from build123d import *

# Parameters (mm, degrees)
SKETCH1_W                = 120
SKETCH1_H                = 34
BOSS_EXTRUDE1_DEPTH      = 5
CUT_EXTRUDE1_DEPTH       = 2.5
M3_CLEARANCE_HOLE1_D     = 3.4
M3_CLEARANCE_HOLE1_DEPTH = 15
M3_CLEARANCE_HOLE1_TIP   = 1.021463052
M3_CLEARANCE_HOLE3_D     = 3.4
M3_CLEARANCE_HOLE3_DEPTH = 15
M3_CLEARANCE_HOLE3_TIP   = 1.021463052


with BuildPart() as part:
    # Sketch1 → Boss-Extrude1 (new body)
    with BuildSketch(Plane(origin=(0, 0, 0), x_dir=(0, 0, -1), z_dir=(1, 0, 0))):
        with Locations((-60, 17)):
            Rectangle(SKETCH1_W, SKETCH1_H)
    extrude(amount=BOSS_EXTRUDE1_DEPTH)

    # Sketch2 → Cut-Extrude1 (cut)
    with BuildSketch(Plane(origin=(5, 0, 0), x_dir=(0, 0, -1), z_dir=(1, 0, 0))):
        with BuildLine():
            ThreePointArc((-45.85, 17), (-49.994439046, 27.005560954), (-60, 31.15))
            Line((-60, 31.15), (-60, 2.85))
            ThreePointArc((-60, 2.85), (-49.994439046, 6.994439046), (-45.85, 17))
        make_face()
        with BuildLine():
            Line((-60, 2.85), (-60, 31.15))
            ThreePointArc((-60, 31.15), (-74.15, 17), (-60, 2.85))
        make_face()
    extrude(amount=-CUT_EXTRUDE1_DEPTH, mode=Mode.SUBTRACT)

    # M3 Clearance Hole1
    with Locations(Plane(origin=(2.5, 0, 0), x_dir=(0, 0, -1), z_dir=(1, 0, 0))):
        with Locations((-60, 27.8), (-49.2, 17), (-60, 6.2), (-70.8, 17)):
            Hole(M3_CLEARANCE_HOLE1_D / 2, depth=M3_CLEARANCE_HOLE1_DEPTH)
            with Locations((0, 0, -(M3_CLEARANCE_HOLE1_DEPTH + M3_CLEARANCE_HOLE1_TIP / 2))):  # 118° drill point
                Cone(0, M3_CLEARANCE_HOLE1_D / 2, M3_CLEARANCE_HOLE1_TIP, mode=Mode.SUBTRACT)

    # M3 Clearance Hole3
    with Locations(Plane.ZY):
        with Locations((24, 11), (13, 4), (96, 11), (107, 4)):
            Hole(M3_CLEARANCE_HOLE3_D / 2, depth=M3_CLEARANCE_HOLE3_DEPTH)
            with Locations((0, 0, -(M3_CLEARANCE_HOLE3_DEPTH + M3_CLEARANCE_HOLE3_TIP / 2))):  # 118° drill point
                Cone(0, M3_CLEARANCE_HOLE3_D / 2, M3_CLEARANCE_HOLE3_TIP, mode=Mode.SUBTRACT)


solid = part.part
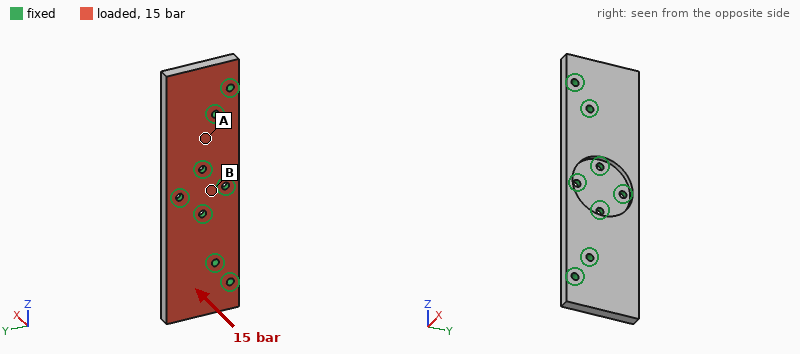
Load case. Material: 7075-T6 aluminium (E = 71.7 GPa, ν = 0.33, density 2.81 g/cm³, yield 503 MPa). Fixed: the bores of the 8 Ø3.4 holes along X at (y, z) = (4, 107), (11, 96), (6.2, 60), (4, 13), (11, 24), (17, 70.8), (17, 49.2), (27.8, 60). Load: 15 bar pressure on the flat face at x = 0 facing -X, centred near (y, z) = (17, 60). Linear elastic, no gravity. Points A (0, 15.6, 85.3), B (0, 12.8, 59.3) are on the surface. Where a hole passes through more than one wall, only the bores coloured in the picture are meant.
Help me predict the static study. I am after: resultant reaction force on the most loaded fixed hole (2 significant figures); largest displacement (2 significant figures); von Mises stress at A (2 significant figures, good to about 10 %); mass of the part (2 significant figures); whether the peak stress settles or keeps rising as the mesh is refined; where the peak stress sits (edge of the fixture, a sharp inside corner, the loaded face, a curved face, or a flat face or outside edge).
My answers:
1.5 kN
0.15 mm
40 MPa
52 g
keeps rising
edge of the fixture
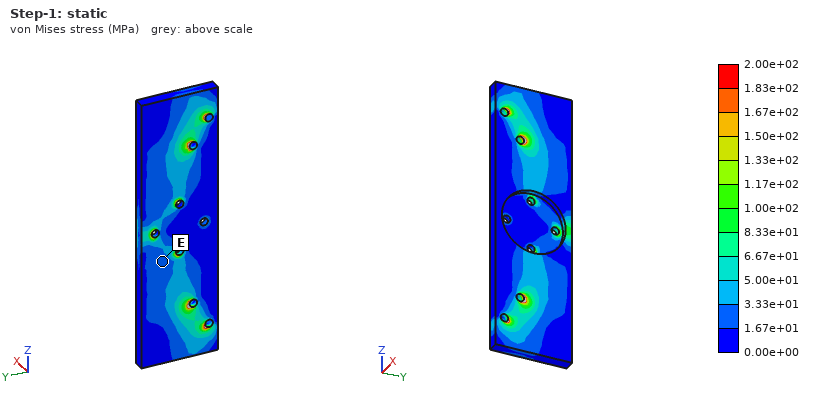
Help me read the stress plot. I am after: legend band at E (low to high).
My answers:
1.67e+01 to 3.33e+01 MPa
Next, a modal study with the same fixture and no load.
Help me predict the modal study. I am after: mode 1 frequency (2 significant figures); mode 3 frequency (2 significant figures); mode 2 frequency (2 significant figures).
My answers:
6000 Hz
10 kHz
6000 Hz
